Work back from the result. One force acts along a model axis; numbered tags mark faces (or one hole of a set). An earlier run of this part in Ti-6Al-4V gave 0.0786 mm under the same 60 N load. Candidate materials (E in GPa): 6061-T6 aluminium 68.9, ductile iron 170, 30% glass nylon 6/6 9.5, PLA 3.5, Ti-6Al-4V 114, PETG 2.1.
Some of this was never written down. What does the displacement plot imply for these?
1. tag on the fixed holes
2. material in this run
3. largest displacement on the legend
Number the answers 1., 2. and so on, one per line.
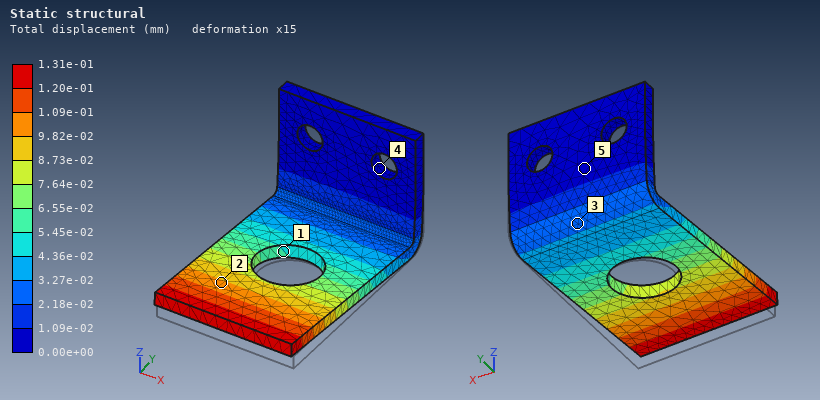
1. 4
2. 6061-T6 aluminium
3. 1.31e-01 mm
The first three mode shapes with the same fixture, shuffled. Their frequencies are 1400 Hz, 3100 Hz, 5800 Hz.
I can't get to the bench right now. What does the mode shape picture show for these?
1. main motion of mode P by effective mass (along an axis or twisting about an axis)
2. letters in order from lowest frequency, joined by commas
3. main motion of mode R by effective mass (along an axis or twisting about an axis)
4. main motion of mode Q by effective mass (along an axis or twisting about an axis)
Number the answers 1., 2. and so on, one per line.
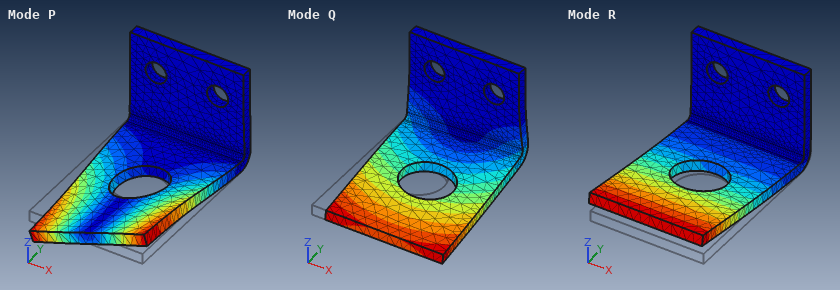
1. twisting about Y
2. R, Q, P
3. along Z
4. along X
